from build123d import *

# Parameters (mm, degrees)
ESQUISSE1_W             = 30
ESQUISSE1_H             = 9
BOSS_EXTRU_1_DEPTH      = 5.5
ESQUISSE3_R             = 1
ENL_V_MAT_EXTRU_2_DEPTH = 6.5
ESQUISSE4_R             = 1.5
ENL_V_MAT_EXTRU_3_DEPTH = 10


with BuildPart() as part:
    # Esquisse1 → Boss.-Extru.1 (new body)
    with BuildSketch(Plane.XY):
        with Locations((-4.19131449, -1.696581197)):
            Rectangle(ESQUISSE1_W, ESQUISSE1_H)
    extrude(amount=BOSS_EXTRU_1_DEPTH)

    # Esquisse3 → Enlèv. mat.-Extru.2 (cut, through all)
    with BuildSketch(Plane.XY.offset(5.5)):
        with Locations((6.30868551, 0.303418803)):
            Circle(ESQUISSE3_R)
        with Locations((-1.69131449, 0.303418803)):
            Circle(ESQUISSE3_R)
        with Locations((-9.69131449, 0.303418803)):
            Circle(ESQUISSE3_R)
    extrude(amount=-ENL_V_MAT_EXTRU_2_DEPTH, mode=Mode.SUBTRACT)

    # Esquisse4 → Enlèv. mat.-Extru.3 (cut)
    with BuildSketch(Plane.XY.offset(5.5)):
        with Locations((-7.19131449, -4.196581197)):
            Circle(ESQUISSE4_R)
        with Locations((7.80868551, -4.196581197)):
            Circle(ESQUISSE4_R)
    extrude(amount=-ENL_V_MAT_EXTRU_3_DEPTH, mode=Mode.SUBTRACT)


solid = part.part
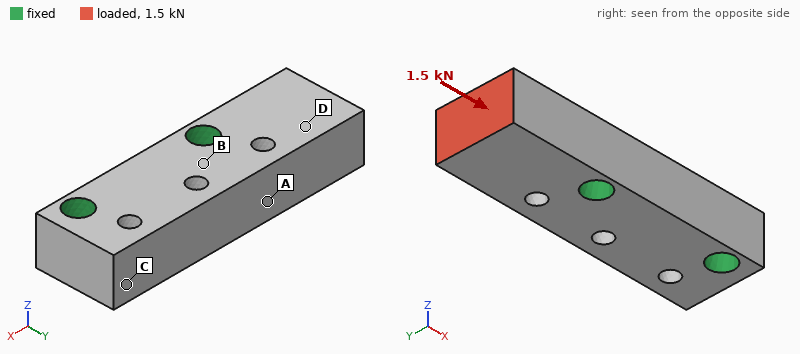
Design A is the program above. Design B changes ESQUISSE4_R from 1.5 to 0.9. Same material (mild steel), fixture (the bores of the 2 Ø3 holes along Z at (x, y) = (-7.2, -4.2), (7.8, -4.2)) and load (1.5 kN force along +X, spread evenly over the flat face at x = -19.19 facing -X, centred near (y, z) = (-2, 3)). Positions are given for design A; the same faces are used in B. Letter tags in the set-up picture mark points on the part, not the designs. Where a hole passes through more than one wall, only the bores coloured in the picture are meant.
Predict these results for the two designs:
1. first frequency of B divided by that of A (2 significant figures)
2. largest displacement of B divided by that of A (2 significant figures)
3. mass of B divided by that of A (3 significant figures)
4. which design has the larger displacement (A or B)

0.88
1.2
1.04
B
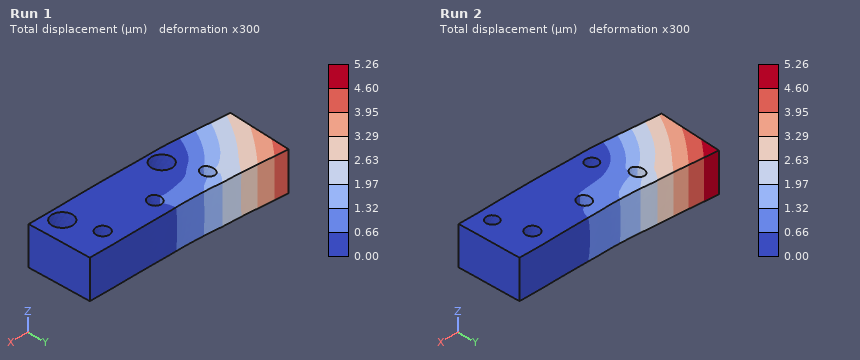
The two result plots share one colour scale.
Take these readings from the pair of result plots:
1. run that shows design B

Run 2
